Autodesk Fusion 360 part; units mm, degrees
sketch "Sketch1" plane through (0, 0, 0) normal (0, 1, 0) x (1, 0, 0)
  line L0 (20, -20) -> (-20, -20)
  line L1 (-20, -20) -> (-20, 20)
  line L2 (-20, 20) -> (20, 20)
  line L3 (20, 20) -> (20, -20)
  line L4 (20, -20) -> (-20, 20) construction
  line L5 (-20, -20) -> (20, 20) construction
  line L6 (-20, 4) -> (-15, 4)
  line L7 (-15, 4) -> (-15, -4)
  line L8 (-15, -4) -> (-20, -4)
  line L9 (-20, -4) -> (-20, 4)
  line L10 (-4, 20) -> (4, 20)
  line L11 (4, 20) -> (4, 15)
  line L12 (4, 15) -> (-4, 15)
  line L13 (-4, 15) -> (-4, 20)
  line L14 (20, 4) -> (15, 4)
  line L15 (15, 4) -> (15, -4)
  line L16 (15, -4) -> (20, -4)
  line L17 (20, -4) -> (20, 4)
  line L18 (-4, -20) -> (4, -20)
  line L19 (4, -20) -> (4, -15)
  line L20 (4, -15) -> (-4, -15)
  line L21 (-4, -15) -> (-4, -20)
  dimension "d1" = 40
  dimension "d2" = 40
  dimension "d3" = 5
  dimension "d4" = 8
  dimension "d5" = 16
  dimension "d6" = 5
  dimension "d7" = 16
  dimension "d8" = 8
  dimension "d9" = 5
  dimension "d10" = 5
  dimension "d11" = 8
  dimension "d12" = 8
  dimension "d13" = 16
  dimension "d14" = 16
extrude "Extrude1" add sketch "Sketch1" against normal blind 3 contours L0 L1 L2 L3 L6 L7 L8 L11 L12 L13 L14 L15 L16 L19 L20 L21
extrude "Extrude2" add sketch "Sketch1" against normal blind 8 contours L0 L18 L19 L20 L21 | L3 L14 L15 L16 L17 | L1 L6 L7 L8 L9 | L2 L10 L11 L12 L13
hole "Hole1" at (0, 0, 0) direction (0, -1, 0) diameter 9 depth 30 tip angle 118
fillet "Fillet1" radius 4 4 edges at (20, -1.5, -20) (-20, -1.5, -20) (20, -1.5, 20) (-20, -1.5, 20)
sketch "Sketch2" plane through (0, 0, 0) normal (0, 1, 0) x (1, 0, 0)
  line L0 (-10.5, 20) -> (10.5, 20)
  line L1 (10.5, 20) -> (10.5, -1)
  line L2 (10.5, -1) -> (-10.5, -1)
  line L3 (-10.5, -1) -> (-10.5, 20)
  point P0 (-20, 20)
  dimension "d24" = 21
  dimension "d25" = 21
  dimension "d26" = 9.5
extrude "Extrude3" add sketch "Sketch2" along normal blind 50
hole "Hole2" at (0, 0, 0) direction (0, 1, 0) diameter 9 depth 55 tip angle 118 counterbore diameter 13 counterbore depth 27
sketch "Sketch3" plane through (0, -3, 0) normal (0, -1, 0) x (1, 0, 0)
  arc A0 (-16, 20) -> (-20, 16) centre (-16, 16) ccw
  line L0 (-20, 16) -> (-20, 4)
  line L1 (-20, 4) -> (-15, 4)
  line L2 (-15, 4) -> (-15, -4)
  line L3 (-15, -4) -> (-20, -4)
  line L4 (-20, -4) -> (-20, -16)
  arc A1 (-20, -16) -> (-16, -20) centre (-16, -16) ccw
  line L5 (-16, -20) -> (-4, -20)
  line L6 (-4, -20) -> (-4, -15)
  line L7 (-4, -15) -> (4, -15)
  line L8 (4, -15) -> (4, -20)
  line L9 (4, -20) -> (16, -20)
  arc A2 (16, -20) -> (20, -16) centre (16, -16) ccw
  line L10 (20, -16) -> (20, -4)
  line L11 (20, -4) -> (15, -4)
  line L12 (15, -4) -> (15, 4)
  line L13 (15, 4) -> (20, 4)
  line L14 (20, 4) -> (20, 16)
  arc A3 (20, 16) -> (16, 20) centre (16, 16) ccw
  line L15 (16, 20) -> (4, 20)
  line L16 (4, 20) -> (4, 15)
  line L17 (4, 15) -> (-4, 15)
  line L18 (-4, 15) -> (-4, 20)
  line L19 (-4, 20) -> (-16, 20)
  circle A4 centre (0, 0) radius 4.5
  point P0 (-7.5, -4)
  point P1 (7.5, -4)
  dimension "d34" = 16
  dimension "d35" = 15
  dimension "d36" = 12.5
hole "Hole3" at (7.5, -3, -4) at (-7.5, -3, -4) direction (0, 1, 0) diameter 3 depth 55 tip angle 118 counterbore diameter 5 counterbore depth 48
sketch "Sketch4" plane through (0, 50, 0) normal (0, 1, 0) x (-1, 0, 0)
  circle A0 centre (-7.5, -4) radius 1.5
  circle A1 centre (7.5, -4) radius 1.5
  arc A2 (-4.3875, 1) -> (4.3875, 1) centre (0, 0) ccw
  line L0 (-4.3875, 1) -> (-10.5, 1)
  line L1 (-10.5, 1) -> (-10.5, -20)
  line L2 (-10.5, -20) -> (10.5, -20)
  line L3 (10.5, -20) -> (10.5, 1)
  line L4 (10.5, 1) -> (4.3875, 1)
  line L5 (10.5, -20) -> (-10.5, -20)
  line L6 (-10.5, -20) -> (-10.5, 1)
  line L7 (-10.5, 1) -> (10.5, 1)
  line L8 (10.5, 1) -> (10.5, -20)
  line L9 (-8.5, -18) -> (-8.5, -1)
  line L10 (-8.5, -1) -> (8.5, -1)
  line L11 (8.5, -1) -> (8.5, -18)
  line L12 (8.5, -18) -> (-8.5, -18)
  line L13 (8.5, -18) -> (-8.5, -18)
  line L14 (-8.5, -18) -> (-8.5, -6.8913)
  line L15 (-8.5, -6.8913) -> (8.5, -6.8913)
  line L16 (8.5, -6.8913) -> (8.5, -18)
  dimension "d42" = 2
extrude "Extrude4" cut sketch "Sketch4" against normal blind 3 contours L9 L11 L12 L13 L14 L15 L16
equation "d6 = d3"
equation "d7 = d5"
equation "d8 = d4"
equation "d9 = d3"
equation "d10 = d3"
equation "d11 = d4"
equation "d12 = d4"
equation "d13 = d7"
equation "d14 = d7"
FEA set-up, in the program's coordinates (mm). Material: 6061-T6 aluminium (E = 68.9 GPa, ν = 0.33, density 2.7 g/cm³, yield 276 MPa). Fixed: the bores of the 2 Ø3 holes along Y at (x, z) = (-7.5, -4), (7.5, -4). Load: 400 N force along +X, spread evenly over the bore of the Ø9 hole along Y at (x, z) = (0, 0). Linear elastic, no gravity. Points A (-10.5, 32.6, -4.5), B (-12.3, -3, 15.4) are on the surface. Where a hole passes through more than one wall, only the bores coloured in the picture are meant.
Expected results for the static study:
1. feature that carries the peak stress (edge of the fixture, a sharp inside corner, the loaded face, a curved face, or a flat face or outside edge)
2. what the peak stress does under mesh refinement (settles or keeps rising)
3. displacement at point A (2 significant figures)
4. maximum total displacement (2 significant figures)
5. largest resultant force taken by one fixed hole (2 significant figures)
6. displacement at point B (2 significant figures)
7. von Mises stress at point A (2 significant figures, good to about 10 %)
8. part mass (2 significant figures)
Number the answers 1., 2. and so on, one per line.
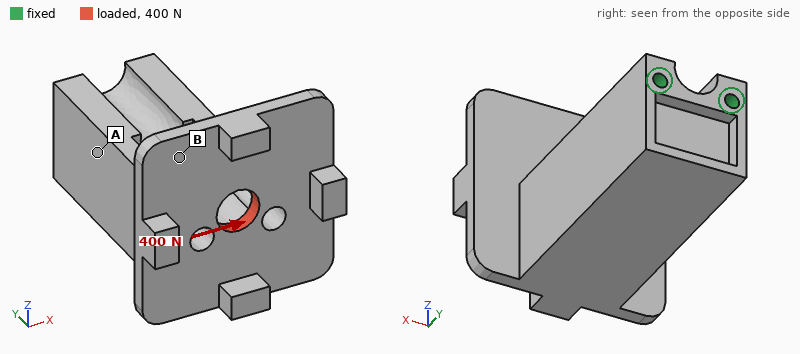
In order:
1. edge of the fixture
2. keeps rising
3. 15 µm
4. 91 µm
5. 1.2 kN
6. 84 µm
7. 18 MPa
8. 59 g
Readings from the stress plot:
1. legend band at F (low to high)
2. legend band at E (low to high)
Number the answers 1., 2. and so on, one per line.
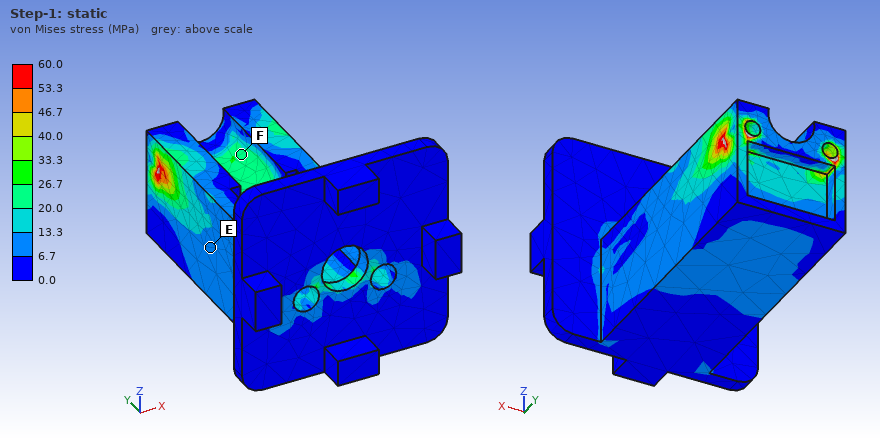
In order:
1. 20.0 to 26.7 MPa
2. 6.7 to 13.3 MPa
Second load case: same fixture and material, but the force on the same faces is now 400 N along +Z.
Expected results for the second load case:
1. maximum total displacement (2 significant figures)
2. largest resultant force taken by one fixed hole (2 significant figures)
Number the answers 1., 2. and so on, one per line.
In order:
1. 0.24 mm
2. 200 N
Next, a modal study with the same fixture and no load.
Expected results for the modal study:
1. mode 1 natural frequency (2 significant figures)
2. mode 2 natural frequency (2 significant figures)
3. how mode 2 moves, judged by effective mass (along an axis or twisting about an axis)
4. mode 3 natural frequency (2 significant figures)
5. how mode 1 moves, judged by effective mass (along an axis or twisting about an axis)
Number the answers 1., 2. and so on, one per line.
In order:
1. 1300 Hz
2. 2600 Hz
3. along X
4. 3900 Hz
5. along Z
